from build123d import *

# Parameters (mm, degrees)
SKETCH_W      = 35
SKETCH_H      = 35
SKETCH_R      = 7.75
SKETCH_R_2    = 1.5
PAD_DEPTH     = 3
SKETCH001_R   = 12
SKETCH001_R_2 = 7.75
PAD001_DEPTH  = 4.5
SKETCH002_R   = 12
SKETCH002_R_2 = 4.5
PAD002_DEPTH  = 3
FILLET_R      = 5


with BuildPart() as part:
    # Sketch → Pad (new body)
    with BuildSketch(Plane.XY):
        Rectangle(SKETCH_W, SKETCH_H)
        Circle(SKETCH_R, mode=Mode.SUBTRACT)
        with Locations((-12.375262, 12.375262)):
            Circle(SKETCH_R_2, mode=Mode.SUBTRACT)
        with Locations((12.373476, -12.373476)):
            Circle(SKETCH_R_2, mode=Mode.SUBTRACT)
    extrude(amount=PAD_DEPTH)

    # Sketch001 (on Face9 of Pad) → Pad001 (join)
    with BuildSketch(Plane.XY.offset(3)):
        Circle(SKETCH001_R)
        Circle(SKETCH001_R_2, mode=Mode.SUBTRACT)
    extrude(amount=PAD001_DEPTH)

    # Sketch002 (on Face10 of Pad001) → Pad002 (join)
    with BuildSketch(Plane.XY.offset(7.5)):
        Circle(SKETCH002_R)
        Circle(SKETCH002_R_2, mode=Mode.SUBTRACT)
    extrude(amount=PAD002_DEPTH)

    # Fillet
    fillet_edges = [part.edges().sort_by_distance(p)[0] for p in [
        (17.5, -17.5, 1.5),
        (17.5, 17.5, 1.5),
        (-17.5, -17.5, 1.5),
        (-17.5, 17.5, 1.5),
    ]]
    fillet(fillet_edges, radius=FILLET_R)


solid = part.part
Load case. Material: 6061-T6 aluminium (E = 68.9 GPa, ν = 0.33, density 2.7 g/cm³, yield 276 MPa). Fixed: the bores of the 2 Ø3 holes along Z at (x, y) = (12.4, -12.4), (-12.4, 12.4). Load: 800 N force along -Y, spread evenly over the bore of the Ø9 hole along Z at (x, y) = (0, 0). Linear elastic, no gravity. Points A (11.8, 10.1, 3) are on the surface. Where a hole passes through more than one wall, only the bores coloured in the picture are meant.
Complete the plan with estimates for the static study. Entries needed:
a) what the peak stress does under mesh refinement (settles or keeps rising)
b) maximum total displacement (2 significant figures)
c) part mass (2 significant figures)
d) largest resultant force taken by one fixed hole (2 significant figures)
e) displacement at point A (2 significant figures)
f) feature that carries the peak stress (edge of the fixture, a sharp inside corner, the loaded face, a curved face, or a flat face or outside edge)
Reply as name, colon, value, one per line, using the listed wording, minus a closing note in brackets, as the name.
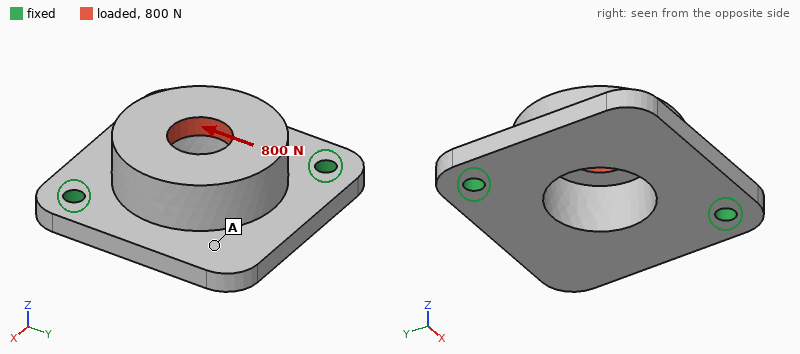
what the peak stress does under mesh refinement: keeps rising
maximum total displacement: 81 µm
part mass: 14 g
largest resultant force taken by one fixed hole: 420 N
displacement at point A: 55 µm
feature that carries the peak stress: edge of the fixture
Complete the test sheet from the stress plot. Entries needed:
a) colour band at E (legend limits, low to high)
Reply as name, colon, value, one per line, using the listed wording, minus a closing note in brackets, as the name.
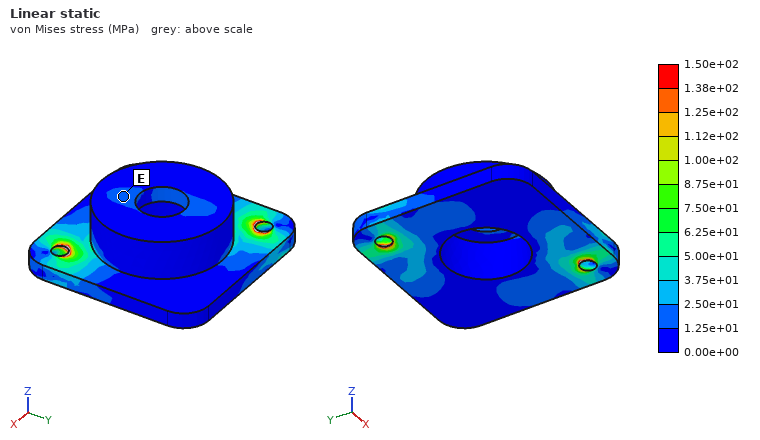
colour band at E: 1.25e+01 to 2.50e+01 MPa
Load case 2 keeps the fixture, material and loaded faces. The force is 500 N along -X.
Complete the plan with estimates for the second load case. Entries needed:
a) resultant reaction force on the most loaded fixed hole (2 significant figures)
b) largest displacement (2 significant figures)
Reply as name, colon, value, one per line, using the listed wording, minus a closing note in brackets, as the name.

resultant reaction force on the most loaded fixed hole: 270 N
largest displacement: 51 µm
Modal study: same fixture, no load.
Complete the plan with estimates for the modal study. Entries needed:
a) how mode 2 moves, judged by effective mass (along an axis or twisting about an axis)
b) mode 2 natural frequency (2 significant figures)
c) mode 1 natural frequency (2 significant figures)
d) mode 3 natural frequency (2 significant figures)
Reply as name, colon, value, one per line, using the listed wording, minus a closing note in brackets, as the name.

how mode 2 moves, judged by effective mass: along Z
mode 2 natural frequency: 10 kHz
mode 1 natural frequency: 4600 Hz
mode 3 natural frequency: 21 kHz
